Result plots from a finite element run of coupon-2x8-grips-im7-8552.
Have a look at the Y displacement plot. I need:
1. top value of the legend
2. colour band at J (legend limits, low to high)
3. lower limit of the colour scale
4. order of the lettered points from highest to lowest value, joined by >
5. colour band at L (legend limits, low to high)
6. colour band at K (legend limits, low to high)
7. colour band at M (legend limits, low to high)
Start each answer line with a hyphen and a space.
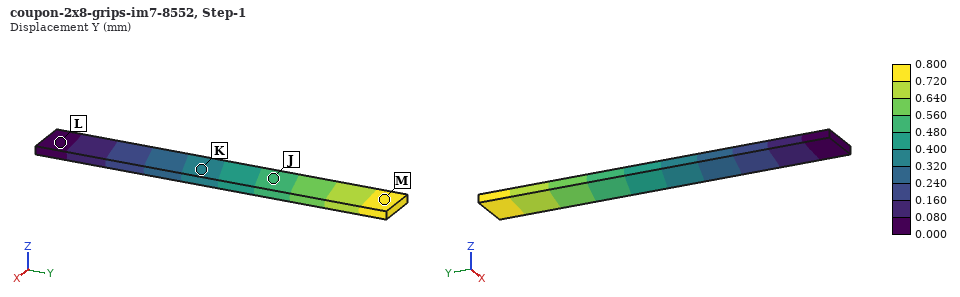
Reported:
- 0.800 mm
- 0.480 to 0.560 mm
- 0.000 mm
- M > J > K > L
- 0.000 to 0.080 mm
- 0.320 to 0.400 mm
- 0.720 to 0.800 mm
